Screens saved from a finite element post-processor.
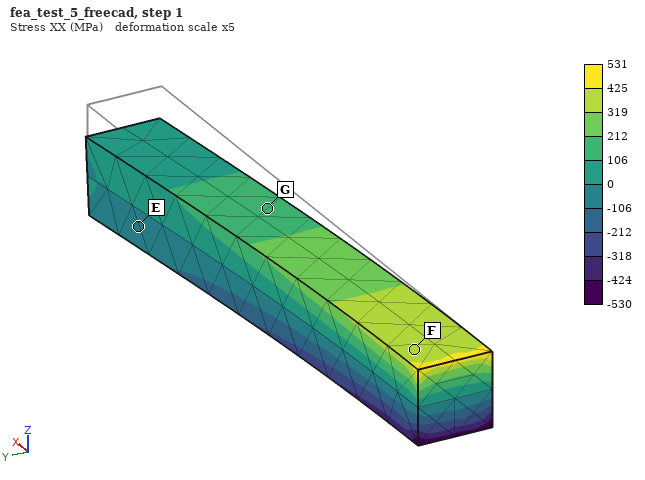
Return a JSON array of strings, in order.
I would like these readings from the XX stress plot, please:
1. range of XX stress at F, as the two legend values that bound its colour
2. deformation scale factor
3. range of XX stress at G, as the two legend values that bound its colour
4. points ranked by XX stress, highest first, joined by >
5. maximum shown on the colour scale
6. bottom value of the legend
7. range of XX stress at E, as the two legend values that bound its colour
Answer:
["319 to 425 MPa", "5", "106 to 212 MPa", "F > G > E", "531 MPa", "-530 MPa", "-106 to 0 MPa"]
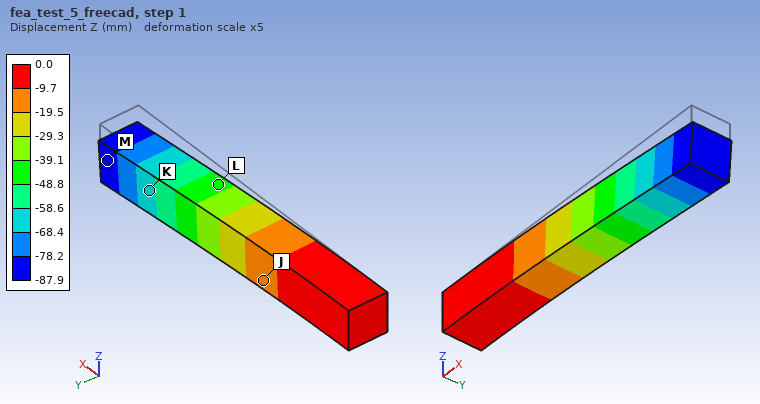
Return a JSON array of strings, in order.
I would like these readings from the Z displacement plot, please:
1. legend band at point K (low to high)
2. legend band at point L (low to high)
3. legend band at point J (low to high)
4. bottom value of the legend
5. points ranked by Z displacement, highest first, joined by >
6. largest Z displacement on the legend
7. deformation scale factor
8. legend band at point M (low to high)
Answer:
["-68.4 to -58.6 mm", "-48.8 to -39.1 mm", "-19.5 to -9.7 mm", "-87.9 mm", "J > L > K > M", "0.0 mm", "5", "-87.9 to -78.2 mm"]
